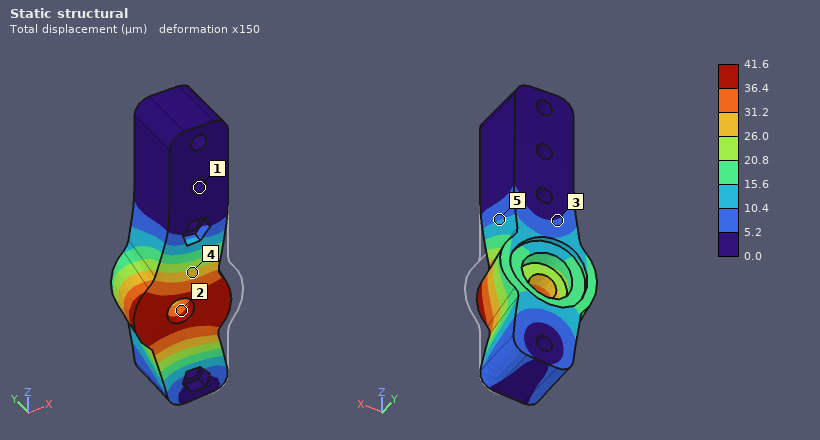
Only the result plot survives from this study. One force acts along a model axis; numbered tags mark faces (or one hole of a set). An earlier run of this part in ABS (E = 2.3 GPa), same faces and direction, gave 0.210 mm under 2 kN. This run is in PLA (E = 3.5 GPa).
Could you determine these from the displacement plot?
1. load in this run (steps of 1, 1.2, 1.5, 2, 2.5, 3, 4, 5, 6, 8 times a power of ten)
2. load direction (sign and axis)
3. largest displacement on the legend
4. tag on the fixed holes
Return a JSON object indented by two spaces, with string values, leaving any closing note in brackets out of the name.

{
  "load in this run": "600 N",
  "load direction": "-X",
  "largest displacement on the legend": "41.6 µm",
  "tag on the fixed holes": "1"
}
